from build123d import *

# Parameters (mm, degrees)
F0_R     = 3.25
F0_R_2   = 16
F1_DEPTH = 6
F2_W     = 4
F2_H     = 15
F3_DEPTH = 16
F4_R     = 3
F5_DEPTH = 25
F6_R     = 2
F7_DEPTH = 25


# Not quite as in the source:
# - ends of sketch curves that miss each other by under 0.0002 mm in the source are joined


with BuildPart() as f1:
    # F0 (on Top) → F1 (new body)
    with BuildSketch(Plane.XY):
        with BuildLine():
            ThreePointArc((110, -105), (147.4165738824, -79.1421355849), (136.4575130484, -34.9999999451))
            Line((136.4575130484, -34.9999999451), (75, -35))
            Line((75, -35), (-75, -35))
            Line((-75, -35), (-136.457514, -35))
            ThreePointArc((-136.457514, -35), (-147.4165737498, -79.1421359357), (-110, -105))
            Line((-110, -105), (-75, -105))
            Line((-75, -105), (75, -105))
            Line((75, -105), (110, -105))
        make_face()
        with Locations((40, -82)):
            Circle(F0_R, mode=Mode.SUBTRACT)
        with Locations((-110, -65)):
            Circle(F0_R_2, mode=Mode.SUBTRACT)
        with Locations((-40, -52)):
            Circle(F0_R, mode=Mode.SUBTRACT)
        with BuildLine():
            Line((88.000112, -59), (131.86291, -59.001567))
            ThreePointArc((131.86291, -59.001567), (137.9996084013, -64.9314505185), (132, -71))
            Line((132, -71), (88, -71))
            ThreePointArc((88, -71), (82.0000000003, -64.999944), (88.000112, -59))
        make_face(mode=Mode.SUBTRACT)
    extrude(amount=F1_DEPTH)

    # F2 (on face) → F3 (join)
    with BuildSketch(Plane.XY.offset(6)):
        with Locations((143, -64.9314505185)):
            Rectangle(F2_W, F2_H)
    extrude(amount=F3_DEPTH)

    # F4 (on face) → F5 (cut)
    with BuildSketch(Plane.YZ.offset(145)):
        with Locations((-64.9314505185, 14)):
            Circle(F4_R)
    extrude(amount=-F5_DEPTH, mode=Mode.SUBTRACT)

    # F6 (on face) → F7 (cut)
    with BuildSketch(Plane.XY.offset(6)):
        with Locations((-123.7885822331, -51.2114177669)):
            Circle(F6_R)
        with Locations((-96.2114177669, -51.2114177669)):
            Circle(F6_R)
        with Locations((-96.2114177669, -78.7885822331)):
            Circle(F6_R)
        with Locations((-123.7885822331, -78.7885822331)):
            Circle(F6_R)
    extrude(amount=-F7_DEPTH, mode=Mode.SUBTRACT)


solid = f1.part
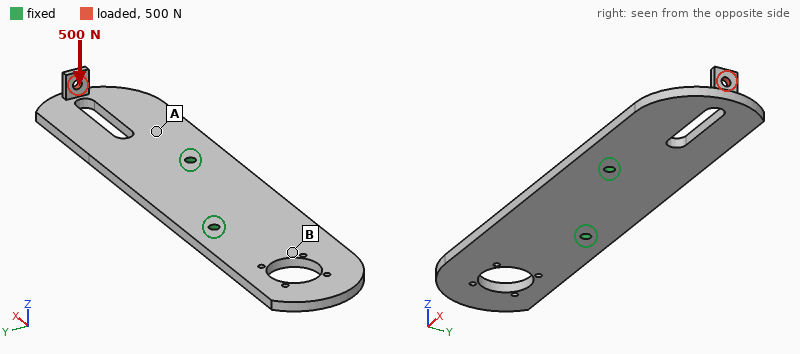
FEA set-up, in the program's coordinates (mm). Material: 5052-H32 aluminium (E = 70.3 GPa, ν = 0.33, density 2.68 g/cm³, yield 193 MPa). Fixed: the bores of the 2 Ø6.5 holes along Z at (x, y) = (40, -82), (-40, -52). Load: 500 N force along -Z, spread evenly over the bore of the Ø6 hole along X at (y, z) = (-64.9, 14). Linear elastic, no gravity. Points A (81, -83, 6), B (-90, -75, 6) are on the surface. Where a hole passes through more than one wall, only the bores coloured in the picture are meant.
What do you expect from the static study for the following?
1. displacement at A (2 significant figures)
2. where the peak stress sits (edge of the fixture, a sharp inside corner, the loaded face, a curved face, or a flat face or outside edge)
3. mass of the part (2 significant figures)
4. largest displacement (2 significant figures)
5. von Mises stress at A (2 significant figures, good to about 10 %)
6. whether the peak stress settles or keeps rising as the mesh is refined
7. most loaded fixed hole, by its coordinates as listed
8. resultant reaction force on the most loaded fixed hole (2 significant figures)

0.50 mm
edge of the fixture
300 g
2.7 mm
76 MPa
keeps rising
(40, -82)
720 N
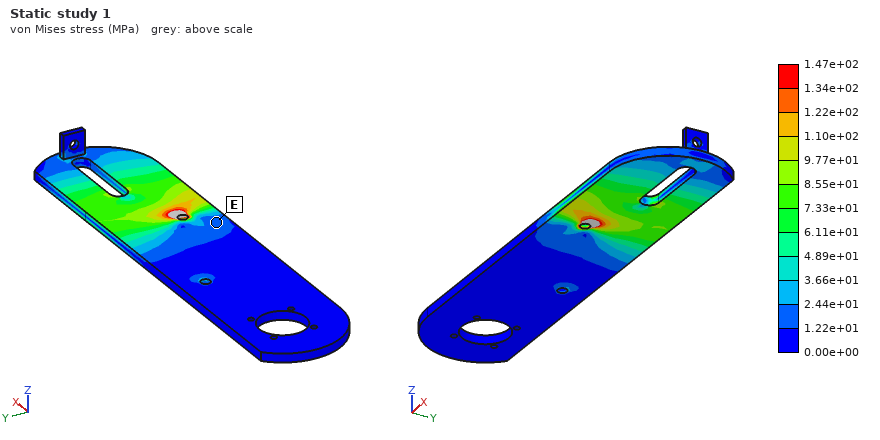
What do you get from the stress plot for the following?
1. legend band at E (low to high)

1.22e+01 to 2.44e+01 MPa
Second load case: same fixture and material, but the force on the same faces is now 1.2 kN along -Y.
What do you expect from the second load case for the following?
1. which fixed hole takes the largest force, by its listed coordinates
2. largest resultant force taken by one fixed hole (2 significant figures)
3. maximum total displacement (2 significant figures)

(40, -82)
2.5 kN
0.53 mm
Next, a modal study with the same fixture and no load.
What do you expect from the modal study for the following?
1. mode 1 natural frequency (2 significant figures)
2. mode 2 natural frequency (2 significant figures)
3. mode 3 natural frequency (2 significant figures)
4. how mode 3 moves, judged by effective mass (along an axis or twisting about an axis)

430 Hz
440 Hz
1100 Hz
twisting about X
